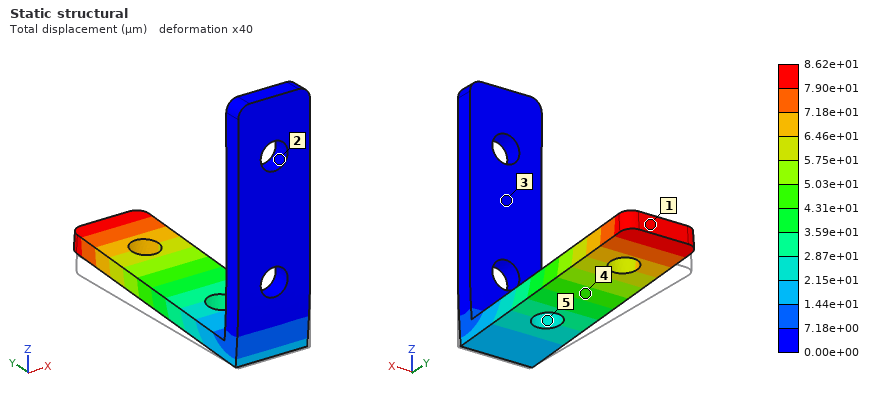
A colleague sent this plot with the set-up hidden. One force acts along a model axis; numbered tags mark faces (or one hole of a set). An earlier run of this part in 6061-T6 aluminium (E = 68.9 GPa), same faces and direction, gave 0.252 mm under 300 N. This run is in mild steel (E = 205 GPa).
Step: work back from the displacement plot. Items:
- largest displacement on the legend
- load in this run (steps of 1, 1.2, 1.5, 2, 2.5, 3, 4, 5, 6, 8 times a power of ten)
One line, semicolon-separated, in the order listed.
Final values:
8.62e+01 µm; 300 N
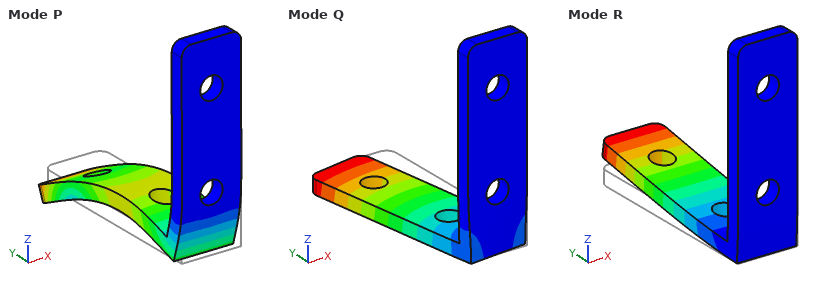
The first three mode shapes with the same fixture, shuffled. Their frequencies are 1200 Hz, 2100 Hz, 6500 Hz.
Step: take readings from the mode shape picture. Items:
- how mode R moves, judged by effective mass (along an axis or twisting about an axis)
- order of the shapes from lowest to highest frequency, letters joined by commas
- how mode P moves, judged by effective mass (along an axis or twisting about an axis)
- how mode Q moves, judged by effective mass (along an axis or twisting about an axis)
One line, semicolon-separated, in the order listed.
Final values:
along Z; R, Q, P; along Y; along X
